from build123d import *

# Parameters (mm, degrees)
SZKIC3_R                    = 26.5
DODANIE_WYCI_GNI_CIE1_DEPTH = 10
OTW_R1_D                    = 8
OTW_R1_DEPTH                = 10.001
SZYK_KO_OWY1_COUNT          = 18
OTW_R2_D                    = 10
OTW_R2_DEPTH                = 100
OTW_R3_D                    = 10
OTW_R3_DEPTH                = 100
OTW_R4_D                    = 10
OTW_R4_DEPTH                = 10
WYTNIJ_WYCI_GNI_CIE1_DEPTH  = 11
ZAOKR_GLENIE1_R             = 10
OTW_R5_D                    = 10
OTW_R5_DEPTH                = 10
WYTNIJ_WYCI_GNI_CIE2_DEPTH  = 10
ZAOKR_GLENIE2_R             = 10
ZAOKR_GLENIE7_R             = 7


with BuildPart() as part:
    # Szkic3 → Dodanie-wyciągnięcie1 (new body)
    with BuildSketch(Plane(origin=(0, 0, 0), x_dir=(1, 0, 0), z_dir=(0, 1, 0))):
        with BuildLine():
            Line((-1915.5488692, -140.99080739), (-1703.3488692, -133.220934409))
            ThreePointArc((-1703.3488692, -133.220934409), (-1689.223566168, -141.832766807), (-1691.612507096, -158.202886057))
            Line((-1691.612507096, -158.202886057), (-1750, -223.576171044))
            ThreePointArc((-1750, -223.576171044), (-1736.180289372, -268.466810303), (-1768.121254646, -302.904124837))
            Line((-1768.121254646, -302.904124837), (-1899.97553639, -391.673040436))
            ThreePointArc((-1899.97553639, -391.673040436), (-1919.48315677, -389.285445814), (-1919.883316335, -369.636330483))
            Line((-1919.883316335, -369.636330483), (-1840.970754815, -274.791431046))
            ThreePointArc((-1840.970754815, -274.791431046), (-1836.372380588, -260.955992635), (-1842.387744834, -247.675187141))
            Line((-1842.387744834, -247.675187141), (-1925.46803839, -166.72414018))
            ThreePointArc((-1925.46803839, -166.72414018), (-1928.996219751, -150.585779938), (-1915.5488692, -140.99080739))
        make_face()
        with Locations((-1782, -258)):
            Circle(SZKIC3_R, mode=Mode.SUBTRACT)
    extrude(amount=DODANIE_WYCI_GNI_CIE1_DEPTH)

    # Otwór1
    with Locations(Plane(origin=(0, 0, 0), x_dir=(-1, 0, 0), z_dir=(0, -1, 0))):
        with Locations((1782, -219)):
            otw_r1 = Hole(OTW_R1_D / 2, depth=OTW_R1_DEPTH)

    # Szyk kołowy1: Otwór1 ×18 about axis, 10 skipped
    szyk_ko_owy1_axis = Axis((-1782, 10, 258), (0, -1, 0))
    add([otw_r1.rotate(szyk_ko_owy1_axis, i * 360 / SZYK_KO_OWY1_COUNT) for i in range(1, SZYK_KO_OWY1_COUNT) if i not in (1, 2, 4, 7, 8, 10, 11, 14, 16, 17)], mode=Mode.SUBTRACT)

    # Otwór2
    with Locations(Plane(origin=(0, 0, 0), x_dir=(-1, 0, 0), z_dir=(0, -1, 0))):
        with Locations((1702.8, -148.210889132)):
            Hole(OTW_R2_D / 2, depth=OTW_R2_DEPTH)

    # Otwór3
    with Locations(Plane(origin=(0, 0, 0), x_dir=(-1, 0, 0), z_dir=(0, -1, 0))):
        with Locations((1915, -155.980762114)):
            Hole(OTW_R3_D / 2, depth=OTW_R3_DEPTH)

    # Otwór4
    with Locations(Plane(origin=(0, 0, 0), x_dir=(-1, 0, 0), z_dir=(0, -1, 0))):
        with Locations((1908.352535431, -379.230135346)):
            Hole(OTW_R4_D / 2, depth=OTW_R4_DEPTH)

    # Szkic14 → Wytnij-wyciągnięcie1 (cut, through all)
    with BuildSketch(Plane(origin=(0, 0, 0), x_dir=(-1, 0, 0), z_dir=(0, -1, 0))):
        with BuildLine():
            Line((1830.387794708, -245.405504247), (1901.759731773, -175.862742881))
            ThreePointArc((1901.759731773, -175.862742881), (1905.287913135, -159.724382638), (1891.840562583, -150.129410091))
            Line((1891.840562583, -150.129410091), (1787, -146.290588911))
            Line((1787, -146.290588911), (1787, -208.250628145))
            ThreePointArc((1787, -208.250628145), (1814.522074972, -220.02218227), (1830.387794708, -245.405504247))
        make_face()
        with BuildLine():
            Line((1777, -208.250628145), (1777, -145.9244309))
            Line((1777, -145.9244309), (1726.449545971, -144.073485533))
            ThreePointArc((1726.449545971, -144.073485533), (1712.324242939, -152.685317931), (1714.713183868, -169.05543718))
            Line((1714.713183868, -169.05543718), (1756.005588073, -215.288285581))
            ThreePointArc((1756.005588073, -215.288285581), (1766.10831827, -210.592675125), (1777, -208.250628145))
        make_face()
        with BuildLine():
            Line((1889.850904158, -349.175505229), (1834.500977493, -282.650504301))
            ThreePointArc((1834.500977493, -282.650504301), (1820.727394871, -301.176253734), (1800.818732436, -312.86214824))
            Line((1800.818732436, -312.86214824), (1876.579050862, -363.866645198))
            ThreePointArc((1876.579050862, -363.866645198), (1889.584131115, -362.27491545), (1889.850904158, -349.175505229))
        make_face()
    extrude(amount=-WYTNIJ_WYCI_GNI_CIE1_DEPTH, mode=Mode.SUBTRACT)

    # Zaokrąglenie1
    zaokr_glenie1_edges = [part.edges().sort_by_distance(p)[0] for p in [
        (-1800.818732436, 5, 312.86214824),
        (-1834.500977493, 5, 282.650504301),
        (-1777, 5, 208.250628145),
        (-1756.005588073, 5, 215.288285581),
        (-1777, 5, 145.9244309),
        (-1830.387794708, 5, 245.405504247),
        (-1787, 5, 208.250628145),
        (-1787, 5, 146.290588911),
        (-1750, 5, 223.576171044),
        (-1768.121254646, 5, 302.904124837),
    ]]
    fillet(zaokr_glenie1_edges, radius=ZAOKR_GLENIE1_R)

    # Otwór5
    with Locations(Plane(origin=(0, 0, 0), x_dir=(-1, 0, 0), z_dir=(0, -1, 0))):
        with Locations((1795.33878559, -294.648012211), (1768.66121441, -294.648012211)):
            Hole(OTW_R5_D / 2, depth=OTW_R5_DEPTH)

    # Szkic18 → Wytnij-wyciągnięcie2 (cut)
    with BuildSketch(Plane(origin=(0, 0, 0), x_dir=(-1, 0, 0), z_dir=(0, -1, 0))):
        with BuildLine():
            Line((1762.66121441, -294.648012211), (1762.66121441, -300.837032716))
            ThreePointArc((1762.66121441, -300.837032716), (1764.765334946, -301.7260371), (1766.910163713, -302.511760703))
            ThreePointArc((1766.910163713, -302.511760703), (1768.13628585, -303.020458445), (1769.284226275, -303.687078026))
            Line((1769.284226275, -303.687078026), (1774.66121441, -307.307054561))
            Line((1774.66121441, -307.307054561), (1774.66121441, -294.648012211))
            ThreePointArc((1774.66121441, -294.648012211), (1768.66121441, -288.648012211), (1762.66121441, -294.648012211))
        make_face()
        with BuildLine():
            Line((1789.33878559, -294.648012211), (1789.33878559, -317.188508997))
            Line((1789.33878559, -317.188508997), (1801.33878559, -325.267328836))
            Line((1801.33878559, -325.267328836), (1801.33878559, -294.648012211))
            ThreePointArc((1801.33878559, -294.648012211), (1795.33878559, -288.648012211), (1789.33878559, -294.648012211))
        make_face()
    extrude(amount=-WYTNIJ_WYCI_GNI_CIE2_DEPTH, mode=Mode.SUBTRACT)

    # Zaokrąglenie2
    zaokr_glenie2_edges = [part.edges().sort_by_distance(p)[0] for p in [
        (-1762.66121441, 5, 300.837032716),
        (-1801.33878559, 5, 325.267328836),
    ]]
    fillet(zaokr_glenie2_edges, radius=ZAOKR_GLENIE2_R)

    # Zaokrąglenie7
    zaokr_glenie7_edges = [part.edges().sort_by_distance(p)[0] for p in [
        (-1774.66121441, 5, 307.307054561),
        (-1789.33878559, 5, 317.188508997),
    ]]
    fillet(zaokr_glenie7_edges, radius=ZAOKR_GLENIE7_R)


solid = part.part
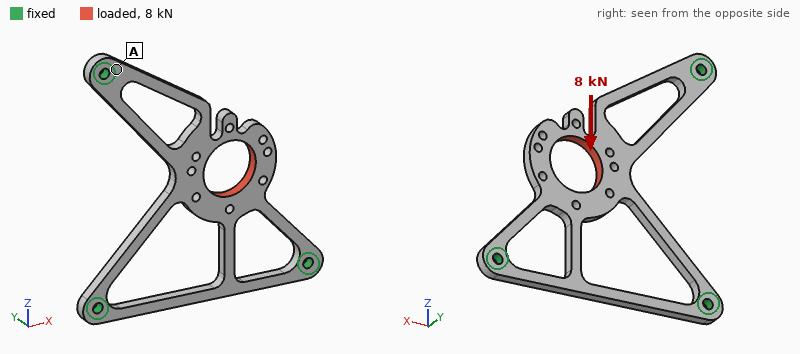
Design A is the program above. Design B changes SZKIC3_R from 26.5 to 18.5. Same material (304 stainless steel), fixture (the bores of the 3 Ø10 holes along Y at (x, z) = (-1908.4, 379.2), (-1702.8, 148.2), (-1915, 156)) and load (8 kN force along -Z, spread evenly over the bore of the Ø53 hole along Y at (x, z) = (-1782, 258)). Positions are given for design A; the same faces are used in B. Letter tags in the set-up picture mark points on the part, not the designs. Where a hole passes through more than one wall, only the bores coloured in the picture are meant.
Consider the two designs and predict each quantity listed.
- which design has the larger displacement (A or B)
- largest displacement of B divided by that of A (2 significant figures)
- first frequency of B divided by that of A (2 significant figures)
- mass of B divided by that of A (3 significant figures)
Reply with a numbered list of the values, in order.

1. A
2. 0.91
3. 0.97
4. 1.08
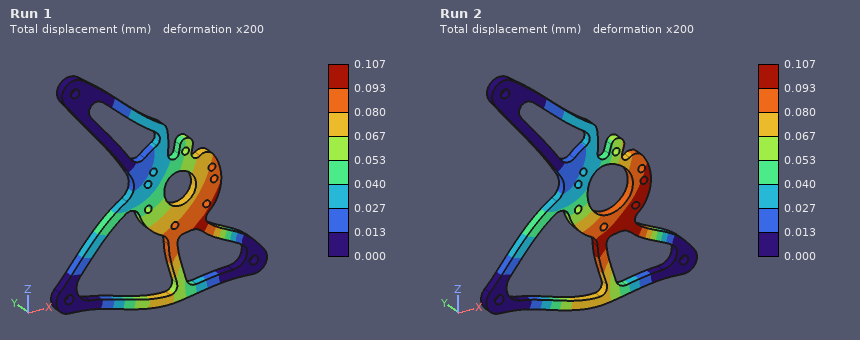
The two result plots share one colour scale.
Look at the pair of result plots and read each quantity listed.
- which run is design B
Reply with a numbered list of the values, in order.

1. Run 1
